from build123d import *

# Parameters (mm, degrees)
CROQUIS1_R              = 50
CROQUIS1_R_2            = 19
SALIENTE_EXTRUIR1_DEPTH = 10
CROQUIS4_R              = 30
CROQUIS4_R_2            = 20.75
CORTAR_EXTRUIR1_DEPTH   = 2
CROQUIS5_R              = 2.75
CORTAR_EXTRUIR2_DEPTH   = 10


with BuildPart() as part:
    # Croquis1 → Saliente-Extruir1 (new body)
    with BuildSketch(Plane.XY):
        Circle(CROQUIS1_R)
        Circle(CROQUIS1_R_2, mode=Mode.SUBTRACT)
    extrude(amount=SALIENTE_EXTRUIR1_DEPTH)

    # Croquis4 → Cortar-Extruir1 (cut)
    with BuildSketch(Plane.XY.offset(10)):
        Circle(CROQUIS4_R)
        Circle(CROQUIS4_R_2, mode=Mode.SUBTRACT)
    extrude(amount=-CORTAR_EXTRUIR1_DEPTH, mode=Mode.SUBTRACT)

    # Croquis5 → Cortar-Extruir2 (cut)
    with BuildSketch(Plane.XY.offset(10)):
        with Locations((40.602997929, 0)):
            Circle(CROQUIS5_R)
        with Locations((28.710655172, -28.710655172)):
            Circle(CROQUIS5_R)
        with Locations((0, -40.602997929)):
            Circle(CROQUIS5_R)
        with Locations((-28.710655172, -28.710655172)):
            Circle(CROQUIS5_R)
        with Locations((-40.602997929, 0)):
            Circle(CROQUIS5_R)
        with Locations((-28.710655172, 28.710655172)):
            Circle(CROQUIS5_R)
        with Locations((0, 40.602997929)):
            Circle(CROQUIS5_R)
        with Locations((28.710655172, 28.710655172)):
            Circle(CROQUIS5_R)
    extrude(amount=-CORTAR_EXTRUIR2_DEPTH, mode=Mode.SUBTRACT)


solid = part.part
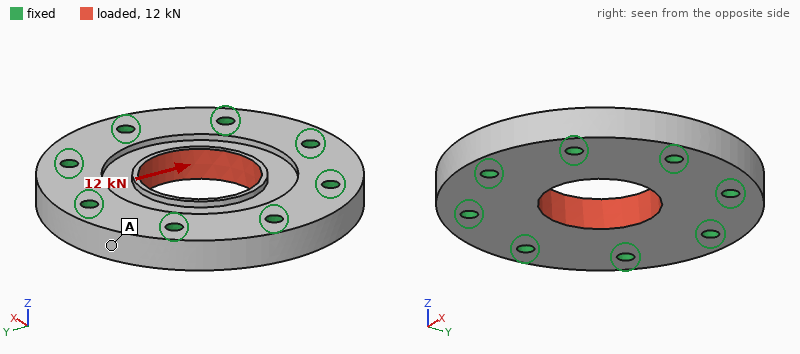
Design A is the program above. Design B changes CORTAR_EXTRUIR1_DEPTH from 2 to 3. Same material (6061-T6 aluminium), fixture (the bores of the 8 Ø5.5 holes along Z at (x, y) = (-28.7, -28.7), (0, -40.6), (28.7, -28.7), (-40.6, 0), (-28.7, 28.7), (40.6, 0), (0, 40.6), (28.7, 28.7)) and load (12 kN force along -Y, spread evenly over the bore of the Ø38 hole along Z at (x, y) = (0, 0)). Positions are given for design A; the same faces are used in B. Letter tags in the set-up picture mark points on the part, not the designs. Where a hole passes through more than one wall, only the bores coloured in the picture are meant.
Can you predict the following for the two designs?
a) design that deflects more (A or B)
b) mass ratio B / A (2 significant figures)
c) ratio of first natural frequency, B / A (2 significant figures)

B
0.98
1.0
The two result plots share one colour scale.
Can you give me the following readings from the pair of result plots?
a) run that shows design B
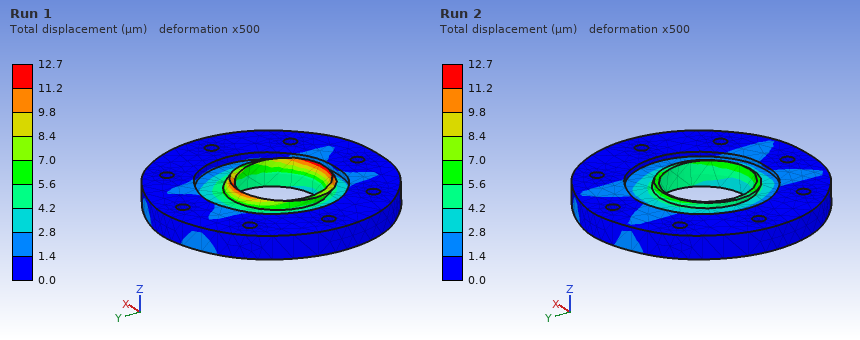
Run 1
